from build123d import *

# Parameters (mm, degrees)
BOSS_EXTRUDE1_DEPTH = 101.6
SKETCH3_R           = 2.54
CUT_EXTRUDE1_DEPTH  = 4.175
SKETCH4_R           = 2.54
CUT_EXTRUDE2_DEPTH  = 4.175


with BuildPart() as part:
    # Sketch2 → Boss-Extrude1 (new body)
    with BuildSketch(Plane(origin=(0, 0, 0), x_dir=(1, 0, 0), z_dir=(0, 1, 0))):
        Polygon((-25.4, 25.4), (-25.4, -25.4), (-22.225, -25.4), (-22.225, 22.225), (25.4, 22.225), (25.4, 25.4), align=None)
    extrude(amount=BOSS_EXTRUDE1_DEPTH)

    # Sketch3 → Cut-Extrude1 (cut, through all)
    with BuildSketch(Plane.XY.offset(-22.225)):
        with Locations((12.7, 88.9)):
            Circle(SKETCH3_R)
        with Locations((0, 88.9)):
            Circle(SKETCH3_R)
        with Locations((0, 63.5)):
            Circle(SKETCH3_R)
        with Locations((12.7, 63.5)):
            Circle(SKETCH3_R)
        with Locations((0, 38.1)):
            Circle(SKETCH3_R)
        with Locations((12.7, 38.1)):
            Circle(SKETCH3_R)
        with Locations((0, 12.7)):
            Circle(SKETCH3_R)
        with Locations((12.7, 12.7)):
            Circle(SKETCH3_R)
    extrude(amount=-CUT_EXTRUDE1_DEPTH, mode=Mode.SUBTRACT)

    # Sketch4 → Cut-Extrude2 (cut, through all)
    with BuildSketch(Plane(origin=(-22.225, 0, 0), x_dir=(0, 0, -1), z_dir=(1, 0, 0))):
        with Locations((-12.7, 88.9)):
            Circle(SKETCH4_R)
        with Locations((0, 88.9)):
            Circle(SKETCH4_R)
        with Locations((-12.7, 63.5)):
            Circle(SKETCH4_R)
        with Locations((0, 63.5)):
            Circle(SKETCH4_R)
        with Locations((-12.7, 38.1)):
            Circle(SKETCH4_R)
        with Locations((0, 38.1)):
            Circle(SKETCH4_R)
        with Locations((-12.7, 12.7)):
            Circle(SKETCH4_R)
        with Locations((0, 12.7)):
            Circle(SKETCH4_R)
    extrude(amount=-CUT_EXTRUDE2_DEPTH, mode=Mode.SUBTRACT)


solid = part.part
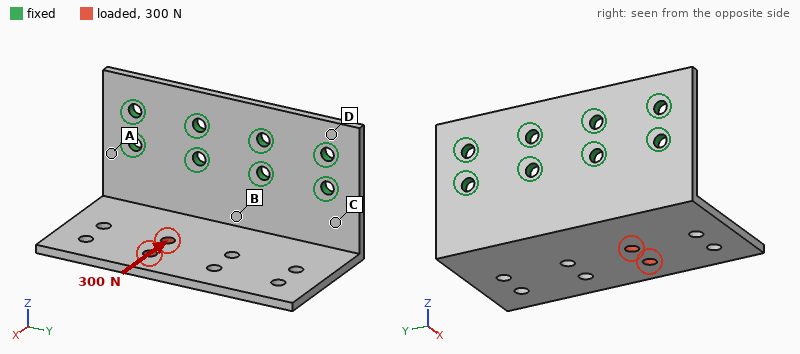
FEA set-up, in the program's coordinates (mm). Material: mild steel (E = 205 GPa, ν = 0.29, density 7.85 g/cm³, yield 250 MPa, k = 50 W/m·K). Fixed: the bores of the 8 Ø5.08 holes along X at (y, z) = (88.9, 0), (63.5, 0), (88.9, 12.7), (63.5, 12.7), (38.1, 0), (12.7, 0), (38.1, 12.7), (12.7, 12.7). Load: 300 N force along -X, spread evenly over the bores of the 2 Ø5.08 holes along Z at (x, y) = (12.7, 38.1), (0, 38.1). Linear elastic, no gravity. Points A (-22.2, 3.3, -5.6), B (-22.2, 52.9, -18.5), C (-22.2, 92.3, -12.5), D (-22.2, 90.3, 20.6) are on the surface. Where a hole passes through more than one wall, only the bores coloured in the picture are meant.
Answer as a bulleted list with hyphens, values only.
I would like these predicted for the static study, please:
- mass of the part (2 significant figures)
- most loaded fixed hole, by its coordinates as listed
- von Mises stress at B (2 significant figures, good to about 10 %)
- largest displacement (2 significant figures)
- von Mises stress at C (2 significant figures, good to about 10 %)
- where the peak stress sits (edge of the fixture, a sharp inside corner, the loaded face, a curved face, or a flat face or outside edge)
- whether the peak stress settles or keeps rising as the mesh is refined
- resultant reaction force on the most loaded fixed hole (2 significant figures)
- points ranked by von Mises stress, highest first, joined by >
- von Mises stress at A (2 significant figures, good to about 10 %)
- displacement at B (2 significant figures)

- 240 g
- (12.7, 0)
- 8.9 MPa
- 86 µm
- 14 MPa
- edge of the fixture
- keeps rising
- 170 N
- A > C > B > D
- 35 MPa
- 15 µm
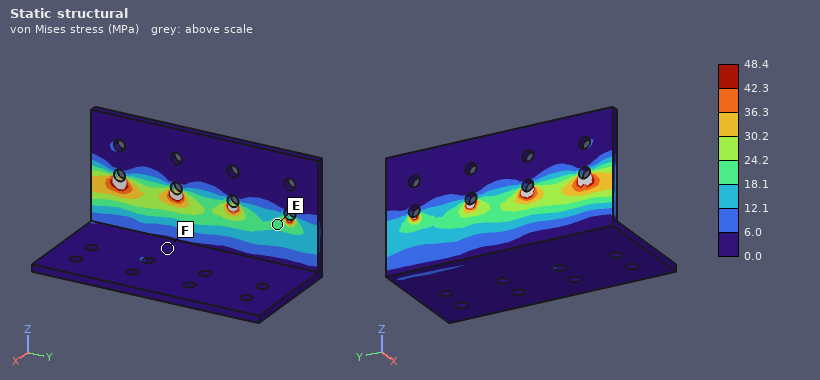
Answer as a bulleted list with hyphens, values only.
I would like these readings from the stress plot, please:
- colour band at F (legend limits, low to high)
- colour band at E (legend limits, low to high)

- 0.0 to 6.0 MPa
- 18.1 to 24.2 MPa
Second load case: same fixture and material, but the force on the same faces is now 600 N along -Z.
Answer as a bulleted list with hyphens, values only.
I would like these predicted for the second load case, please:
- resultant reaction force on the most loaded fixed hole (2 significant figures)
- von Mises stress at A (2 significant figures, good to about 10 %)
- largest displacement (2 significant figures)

- 230 N
- 110 MPa
- 0.60 mm
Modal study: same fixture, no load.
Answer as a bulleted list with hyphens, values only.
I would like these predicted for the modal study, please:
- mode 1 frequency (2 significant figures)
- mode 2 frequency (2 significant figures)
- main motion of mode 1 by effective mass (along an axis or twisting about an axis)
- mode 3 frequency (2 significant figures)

- 650 Hz
- 1200 Hz
- along Z
- 2000 Hz
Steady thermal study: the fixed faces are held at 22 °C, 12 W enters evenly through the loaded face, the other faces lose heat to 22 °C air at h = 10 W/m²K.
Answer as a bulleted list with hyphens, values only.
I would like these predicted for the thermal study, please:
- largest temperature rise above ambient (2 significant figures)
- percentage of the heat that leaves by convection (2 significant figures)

- 51 K
- 26 %
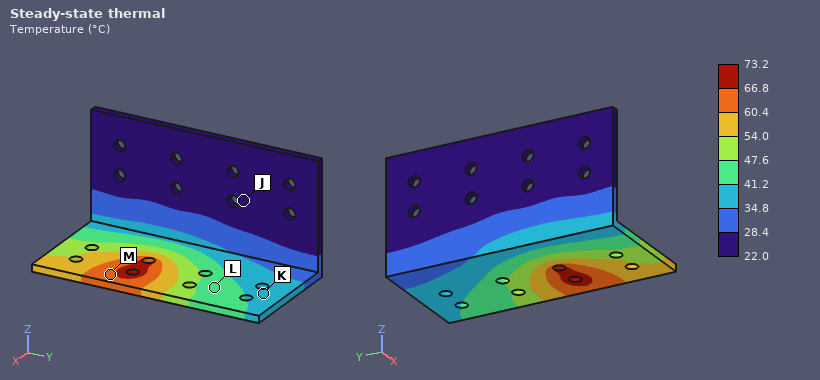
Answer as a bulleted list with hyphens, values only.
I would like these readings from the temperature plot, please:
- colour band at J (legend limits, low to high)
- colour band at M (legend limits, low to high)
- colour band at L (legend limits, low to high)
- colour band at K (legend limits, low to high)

- 22.0 to 28.4 °C
- 60.4 to 66.8 °C
- 41.2 to 47.6 °C
- 34.8 to 41.2 °C
